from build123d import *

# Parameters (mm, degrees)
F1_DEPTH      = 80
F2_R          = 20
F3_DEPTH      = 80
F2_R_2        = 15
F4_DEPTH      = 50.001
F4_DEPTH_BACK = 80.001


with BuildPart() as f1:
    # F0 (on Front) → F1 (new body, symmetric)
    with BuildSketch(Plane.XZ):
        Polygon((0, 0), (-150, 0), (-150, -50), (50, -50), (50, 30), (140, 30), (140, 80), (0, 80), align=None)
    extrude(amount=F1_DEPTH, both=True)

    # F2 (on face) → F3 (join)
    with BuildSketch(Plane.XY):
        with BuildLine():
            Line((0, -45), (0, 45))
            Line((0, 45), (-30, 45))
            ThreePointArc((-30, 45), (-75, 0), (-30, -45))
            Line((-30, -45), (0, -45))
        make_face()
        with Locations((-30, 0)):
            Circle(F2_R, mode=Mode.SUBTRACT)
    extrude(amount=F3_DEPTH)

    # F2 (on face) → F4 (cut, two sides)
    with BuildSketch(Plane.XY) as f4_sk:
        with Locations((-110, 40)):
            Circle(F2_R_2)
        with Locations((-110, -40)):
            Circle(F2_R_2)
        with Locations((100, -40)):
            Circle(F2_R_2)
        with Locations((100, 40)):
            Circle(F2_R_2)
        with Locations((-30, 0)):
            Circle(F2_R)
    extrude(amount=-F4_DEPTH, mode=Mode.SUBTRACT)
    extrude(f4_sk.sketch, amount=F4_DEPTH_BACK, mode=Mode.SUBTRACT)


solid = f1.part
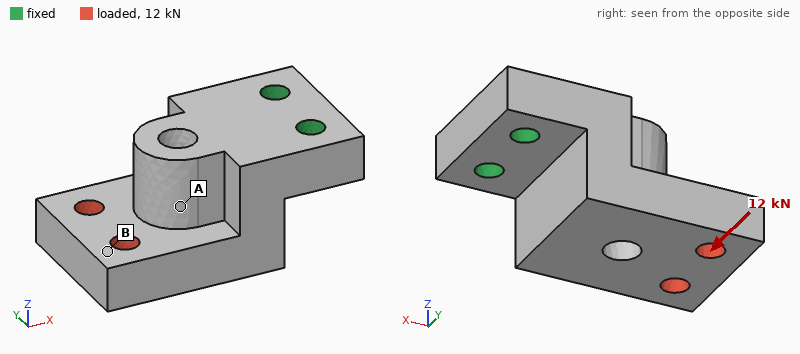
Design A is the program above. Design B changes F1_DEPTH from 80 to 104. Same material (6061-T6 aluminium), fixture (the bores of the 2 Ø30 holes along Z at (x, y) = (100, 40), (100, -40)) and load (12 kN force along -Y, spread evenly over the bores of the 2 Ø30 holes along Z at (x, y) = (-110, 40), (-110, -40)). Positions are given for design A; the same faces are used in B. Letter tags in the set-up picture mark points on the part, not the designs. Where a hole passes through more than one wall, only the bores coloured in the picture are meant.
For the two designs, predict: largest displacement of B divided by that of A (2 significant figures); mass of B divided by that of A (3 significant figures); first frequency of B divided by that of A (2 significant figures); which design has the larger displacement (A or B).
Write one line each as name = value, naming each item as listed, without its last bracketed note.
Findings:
largest displacement of B divided by that of A = 0.76
mass of B divided by that of A = 1.28
first frequency of B divided by that of A = 0.95
which design has the larger displacement = A
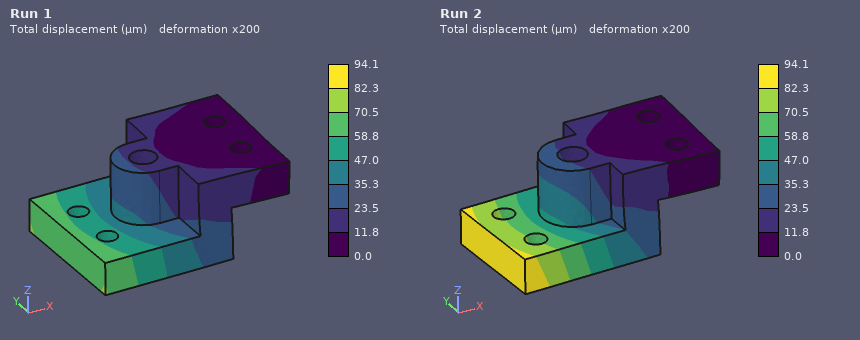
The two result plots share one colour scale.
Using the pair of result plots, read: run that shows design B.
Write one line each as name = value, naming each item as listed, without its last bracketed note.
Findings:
run that shows design B = Run 1
